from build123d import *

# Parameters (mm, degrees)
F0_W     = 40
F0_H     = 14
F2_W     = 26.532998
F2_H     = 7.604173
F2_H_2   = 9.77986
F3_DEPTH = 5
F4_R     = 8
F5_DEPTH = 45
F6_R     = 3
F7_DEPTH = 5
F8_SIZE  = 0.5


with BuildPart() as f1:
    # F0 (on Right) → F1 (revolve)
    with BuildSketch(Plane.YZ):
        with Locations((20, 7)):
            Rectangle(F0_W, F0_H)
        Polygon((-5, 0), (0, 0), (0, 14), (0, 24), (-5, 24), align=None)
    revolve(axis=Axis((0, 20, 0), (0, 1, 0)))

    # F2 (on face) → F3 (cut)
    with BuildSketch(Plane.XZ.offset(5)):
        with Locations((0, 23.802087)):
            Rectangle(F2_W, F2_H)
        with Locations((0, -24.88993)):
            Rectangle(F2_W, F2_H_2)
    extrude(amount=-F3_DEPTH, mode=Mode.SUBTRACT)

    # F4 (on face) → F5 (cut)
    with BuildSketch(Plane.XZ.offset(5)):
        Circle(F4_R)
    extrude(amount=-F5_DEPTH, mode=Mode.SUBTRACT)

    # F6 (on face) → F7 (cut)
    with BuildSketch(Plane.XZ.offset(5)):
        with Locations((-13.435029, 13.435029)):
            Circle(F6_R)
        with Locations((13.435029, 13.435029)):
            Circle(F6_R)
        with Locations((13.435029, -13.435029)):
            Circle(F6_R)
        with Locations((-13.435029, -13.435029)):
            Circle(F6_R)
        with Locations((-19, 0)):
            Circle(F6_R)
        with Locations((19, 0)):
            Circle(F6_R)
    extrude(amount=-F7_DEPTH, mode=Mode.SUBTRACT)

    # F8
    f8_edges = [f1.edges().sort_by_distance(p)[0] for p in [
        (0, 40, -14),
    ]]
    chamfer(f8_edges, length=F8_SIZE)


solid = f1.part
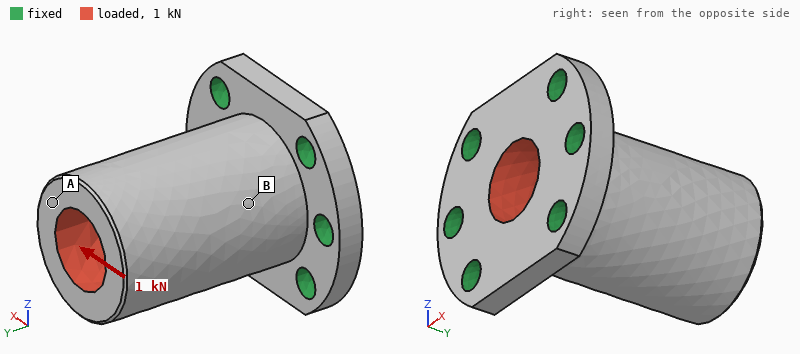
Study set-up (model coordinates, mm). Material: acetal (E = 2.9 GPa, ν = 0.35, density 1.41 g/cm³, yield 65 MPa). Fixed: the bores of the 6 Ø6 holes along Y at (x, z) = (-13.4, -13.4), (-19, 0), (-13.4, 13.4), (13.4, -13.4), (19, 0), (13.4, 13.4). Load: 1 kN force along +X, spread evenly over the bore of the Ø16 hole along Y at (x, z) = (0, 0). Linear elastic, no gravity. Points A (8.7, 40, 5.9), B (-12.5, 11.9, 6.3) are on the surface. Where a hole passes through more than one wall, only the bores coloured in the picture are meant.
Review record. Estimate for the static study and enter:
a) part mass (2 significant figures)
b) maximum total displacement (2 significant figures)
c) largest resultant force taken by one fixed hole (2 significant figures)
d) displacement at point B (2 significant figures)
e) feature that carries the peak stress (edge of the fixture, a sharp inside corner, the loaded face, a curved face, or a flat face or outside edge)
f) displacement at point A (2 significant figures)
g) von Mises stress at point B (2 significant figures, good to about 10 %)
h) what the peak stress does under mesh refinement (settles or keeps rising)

33 g
0.26 mm
390 N
0.097 mm
edge of the fixture
0.26 mm
3.9 MPa
keeps rising
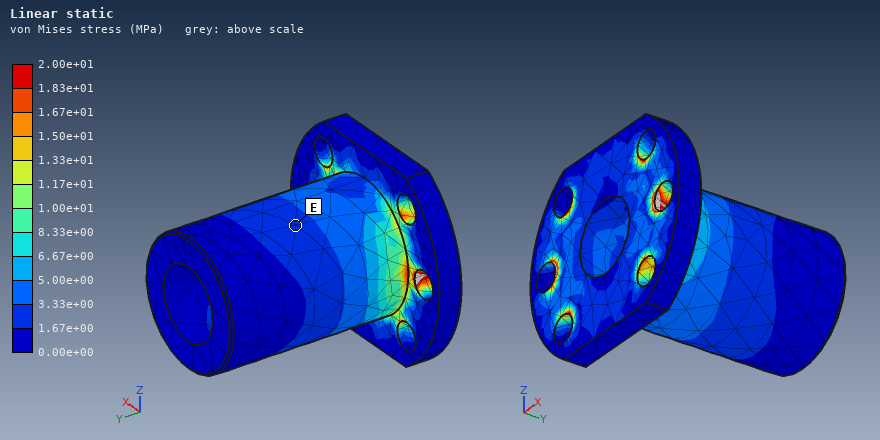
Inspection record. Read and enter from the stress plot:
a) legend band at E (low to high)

1.67e+00 to 3.33e+00 MPa
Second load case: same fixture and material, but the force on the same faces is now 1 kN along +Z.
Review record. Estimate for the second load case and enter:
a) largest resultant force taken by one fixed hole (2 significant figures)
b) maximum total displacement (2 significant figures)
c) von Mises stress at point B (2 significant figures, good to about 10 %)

480 N
0.35 mm
3.7 MPa
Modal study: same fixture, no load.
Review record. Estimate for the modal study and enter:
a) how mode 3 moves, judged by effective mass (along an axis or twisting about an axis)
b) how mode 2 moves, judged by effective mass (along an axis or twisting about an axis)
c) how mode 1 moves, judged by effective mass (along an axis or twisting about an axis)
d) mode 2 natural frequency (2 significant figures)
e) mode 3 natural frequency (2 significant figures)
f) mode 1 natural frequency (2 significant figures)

twisting about Y
along X
along Z
2300 Hz
5000 Hz
2000 Hz
